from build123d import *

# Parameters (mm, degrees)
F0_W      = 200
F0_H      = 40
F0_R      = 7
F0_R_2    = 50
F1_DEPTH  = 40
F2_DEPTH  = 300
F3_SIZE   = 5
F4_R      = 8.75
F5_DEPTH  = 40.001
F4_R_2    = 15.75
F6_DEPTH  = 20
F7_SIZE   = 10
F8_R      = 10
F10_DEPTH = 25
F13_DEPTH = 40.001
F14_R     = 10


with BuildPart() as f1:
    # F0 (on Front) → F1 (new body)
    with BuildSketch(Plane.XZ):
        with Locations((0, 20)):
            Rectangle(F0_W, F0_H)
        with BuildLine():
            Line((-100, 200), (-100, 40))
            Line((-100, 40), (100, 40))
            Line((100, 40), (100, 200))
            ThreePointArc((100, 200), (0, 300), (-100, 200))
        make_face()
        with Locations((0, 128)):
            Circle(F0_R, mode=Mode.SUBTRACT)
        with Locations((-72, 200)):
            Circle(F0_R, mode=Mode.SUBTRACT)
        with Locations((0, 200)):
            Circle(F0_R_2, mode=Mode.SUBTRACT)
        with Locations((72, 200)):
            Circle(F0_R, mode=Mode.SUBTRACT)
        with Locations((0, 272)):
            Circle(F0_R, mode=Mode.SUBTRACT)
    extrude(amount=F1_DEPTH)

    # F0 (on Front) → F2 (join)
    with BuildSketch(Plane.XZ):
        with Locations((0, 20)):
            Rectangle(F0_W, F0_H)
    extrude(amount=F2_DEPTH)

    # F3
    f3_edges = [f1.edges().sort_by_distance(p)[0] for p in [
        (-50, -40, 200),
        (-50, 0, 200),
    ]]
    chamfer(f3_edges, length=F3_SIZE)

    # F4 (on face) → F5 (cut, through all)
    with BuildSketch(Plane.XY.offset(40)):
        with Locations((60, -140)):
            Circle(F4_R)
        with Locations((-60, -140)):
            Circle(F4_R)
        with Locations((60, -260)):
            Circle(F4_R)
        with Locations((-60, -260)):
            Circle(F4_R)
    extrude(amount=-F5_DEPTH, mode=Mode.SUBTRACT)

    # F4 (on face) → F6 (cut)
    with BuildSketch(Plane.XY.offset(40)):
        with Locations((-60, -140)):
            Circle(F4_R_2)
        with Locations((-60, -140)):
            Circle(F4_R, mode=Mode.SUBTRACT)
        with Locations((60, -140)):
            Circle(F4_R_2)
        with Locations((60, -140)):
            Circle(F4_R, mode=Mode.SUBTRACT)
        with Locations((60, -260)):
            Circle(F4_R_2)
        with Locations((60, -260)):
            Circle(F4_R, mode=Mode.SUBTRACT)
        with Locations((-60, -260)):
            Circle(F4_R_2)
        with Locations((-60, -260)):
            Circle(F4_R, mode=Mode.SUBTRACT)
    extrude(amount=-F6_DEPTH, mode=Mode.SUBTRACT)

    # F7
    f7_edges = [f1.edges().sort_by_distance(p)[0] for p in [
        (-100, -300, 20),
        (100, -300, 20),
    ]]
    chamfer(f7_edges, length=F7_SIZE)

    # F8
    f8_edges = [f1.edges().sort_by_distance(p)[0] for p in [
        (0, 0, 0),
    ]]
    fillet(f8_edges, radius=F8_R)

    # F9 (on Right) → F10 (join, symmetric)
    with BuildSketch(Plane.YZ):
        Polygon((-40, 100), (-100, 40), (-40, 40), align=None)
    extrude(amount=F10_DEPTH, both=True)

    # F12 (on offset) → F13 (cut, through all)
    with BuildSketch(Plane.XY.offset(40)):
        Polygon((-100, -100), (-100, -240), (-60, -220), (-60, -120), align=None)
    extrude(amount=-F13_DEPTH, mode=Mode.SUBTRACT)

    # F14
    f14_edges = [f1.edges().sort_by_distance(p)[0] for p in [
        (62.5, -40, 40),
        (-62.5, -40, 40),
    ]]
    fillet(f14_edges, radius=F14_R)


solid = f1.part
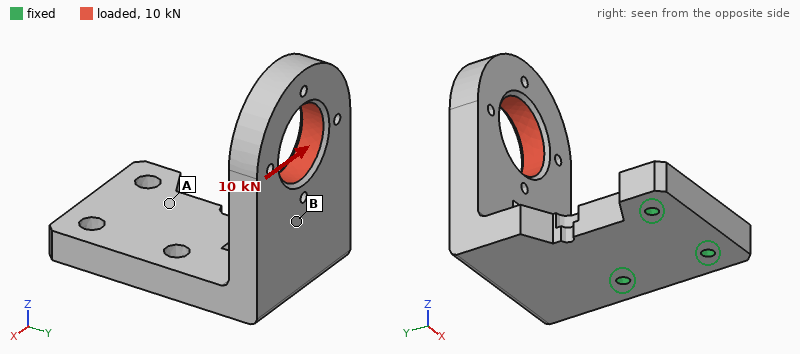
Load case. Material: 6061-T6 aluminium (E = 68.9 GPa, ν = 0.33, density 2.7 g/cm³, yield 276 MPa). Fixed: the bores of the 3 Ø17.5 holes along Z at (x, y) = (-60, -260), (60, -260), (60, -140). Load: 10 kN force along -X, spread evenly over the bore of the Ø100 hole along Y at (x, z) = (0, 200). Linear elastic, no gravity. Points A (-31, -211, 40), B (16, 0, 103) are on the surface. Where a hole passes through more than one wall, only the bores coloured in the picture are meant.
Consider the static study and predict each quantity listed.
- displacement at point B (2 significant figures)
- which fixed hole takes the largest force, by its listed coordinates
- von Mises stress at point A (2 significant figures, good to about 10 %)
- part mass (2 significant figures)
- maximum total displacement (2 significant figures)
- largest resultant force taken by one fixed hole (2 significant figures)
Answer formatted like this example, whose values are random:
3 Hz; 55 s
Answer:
0.36 mm; (-60, -260); 30 MPa; 10 kg; 1.0 mm; 21 kN
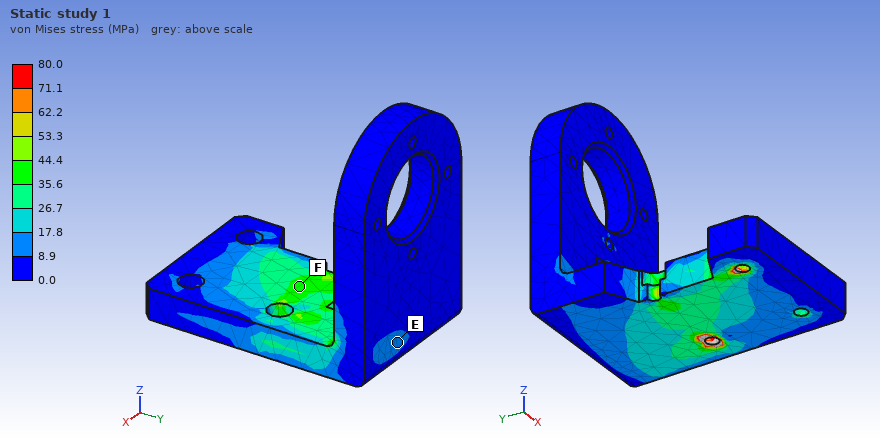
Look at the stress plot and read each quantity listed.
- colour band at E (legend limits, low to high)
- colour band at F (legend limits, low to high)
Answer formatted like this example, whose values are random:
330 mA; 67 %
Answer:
8.9 to 17.8 MPa; 35.6 to 44.4 MPa
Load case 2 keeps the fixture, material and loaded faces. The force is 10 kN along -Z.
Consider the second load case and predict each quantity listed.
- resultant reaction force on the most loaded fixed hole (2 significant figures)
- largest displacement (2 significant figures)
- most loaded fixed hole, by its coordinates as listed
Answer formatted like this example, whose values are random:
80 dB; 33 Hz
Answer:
18 kN; 0.73 mm; (60, -140)
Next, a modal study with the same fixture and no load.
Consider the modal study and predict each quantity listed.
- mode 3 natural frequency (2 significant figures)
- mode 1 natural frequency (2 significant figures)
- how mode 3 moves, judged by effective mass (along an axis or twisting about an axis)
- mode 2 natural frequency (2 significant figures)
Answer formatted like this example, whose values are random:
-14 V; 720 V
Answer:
880 Hz; 250 Hz; along Z; 370 Hz
